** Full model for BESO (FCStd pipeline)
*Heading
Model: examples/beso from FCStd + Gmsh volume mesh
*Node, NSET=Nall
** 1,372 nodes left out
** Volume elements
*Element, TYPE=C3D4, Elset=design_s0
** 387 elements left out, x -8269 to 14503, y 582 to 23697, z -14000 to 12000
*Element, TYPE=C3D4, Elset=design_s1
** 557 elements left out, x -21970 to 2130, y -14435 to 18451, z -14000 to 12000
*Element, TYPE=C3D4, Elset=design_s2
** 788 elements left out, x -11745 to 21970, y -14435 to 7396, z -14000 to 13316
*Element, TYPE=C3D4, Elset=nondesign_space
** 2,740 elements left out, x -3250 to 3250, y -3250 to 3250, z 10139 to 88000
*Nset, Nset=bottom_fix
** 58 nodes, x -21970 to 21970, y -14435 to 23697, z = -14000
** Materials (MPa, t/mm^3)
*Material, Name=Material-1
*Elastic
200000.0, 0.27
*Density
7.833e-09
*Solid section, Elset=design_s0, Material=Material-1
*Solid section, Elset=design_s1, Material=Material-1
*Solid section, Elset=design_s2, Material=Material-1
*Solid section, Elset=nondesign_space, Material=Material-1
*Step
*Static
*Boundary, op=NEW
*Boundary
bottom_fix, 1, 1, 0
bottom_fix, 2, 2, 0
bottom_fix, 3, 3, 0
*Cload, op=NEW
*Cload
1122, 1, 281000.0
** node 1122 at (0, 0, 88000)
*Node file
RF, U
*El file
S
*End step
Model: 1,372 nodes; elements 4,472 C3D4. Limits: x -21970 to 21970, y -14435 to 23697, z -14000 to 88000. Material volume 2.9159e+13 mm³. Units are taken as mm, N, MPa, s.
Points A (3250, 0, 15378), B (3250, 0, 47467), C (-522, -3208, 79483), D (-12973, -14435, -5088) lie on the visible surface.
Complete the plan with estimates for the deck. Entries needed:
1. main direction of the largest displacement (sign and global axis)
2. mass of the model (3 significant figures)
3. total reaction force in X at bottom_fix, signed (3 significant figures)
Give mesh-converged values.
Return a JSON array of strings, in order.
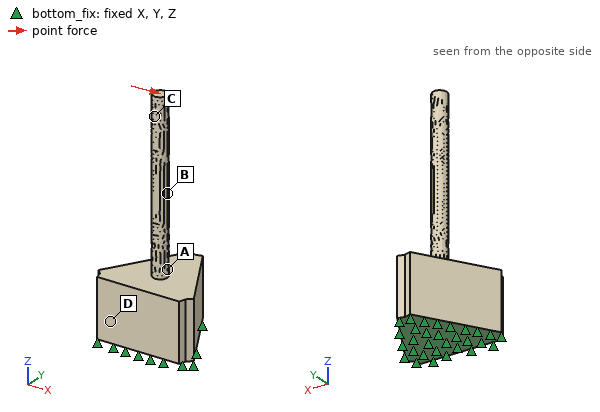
["+X", "2.28e+08 kg", "-2.81e+05 N"]
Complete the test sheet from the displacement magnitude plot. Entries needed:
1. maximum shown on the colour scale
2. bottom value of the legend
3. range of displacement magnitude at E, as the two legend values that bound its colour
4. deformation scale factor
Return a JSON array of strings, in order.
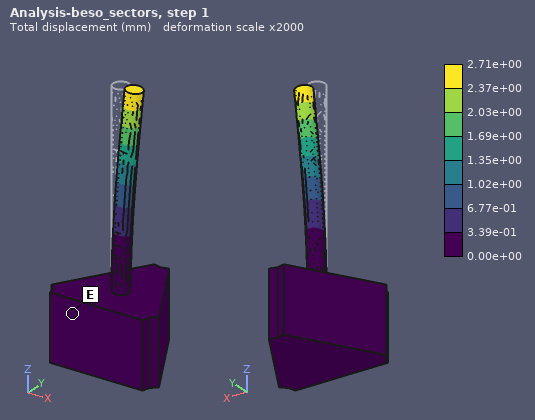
["2.71e+00 mm", "0.00e+00 mm", "0.00e+00 to 3.39e-01 mm", "2000"]
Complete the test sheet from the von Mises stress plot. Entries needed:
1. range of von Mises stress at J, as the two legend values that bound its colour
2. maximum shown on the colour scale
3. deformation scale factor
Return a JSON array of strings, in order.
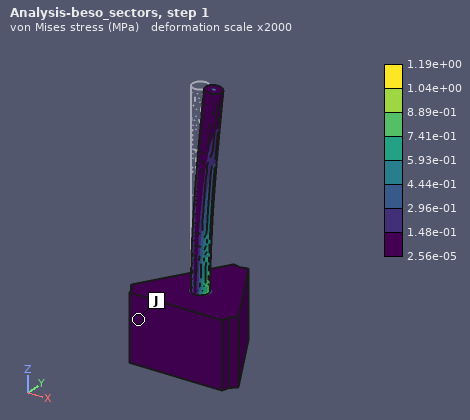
["2.56e-05 to 1.48e-01 MPa", "1.19e+00 MPa", "2000"]
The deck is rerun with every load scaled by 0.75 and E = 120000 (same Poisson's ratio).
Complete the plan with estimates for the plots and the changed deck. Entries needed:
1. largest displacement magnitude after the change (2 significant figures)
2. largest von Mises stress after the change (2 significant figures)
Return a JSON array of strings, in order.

["3.4 mm", "0.89 MPa"]
